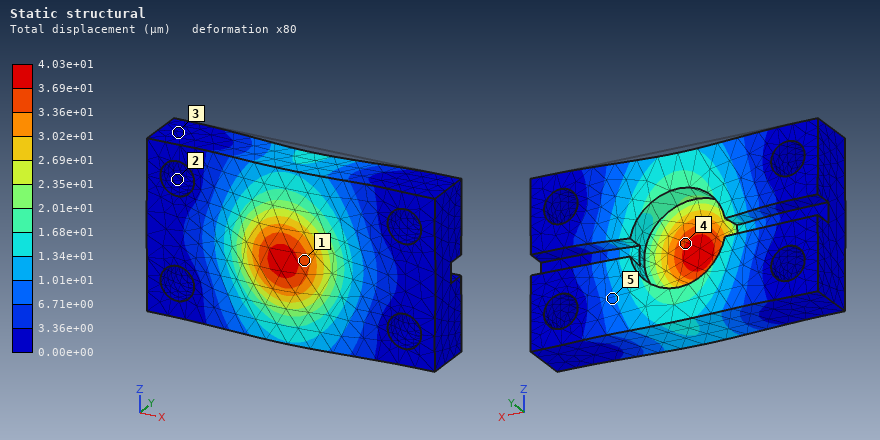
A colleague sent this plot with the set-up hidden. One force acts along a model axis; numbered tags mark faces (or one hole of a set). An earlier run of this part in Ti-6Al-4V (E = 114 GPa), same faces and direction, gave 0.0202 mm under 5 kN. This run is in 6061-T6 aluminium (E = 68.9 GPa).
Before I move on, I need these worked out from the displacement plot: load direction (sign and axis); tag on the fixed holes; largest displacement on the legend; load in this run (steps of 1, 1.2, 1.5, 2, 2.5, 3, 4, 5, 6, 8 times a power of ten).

-Y
2
4.03e+01 µm
6 kN
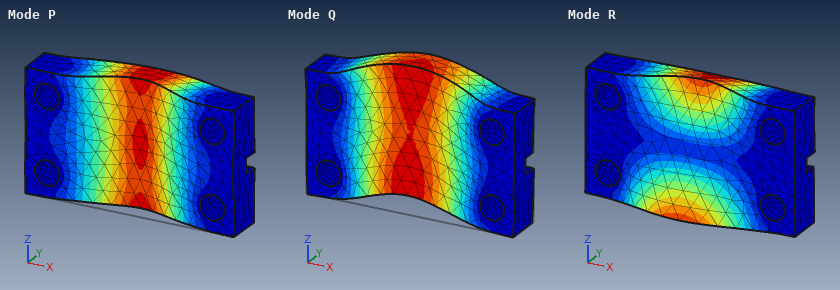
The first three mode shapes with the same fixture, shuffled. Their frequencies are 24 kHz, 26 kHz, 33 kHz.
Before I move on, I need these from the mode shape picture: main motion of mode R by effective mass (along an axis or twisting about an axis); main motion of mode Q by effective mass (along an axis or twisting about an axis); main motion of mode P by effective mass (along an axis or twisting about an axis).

twisting about X
along Z
along Y
